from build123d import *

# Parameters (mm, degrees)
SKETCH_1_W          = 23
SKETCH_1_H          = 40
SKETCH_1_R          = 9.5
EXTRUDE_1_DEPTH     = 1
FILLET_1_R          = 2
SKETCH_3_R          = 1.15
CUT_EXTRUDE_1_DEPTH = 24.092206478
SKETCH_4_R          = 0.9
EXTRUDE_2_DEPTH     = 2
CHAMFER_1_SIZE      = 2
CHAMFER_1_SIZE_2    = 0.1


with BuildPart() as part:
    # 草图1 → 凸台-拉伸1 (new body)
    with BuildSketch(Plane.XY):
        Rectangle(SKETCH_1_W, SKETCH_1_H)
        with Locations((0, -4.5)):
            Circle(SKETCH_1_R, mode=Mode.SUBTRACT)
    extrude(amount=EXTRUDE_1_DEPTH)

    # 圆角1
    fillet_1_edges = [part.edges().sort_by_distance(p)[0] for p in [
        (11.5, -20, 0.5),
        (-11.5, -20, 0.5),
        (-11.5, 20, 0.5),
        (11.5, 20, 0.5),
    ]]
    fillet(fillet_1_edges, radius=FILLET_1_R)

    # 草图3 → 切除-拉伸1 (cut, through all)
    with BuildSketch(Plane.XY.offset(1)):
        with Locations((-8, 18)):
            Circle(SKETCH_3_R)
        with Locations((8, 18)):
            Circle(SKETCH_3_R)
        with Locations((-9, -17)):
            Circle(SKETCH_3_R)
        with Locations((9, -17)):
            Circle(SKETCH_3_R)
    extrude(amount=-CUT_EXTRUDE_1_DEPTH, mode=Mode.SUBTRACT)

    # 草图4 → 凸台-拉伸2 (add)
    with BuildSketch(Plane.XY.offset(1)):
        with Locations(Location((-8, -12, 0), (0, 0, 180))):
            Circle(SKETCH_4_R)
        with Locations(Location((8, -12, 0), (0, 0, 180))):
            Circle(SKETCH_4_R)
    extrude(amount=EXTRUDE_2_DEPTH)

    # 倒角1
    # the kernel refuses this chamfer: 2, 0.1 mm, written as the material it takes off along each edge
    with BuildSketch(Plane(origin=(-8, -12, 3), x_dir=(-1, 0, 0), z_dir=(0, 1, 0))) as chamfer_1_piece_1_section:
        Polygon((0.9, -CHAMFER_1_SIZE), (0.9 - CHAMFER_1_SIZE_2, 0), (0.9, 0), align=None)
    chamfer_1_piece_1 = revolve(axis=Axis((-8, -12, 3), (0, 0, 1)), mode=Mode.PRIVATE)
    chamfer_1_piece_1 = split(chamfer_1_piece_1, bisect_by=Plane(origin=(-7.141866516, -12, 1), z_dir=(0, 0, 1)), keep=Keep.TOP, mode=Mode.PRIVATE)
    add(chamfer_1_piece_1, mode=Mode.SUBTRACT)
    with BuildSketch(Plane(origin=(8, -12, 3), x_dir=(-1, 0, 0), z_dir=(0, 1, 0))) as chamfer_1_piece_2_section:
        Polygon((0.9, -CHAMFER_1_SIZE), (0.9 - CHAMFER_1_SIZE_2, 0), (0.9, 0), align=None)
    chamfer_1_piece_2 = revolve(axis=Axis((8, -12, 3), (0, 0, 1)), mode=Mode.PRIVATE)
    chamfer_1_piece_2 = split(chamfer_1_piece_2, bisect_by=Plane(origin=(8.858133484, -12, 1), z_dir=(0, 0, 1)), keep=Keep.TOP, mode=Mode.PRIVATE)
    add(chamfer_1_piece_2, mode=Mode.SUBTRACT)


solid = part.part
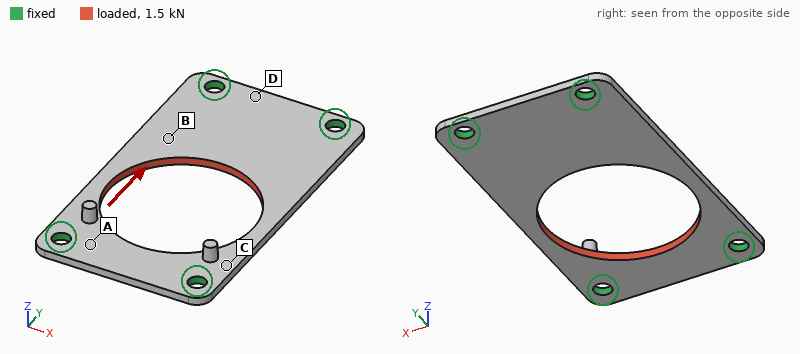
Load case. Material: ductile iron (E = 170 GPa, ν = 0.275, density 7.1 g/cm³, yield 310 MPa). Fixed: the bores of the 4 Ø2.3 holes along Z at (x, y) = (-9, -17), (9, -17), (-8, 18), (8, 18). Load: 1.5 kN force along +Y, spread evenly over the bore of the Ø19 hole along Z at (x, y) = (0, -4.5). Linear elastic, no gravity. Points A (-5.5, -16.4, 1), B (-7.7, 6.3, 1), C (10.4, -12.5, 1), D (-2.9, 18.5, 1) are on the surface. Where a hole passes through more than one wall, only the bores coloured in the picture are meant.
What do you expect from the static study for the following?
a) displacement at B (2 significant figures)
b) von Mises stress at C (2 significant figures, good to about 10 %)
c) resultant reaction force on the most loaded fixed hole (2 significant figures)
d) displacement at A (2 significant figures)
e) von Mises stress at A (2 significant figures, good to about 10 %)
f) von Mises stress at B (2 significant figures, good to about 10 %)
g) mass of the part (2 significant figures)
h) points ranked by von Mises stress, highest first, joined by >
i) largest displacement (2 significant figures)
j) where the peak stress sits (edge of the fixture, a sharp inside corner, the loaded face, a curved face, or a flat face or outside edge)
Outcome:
2.7 µm
62 MPa
430 N
2.4 µm
46 MPa
32 MPa
4.4 g
C > A > B > D
5.1 µm
edge of the fixture
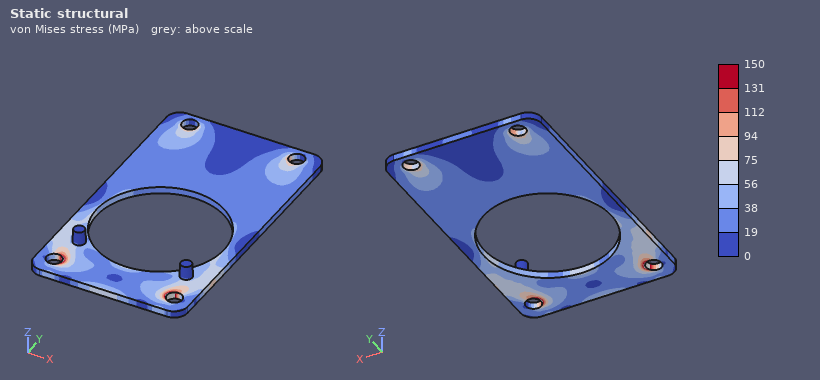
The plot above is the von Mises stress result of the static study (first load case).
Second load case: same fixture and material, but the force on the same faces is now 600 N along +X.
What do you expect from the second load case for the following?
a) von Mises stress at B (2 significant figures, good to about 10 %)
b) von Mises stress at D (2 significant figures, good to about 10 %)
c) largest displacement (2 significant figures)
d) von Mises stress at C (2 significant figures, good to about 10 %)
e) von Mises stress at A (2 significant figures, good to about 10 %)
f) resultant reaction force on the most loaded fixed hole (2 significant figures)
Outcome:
16 MPa
11 MPa
9.5 µm
10 MPa
30 MPa
220 N
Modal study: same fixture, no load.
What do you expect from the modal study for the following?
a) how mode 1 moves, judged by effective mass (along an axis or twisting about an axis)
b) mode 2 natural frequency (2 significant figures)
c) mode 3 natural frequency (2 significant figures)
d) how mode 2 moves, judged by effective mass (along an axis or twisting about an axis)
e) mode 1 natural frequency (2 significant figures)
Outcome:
along Z
6000 Hz
11 kHz
twisting about Y
4600 Hz
